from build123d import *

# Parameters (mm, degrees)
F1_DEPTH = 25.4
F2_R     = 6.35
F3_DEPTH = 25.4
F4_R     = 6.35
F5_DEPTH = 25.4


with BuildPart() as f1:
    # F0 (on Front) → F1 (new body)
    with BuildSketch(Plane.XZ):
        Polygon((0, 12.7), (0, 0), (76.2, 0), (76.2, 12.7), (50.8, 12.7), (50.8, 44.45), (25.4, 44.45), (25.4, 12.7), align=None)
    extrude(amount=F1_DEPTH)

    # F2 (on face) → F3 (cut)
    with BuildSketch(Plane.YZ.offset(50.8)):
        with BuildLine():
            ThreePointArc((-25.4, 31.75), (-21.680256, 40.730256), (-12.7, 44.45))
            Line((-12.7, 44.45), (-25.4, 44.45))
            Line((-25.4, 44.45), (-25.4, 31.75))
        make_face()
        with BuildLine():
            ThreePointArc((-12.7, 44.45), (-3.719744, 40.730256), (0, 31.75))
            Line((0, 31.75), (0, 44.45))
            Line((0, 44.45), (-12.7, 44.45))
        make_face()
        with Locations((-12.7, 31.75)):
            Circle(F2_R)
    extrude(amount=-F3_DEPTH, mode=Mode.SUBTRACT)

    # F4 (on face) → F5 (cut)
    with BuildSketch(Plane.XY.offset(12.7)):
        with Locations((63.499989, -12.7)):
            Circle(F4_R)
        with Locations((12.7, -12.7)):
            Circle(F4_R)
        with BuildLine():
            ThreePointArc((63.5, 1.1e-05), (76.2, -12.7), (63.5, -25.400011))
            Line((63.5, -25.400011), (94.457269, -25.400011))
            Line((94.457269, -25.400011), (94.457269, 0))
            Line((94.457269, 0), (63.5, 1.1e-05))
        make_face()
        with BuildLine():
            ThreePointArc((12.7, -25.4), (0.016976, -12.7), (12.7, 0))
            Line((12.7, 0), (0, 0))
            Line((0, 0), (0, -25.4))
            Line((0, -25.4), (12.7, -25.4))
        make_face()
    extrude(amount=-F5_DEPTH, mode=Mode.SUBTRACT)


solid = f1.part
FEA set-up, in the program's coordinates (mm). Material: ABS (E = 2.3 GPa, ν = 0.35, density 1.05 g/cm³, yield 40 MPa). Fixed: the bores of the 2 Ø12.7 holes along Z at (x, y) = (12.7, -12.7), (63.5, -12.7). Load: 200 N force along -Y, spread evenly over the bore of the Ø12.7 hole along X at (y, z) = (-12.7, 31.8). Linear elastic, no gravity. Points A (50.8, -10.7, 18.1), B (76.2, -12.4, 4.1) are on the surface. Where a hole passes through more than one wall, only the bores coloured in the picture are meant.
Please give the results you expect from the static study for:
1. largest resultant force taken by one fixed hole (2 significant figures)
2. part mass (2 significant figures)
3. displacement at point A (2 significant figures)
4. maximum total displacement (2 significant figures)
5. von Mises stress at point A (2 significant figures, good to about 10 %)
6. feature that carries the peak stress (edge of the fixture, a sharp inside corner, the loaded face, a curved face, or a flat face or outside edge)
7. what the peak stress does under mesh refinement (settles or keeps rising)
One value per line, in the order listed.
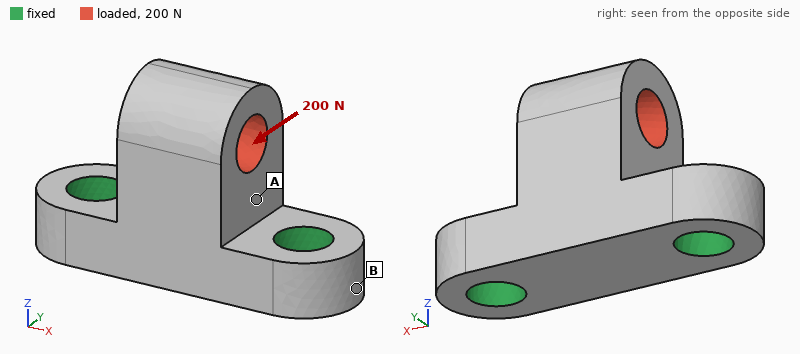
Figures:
100 N
37 g
0.038 mm
0.13 mm
1.4 MPa
edge of the fixture
keeps rising
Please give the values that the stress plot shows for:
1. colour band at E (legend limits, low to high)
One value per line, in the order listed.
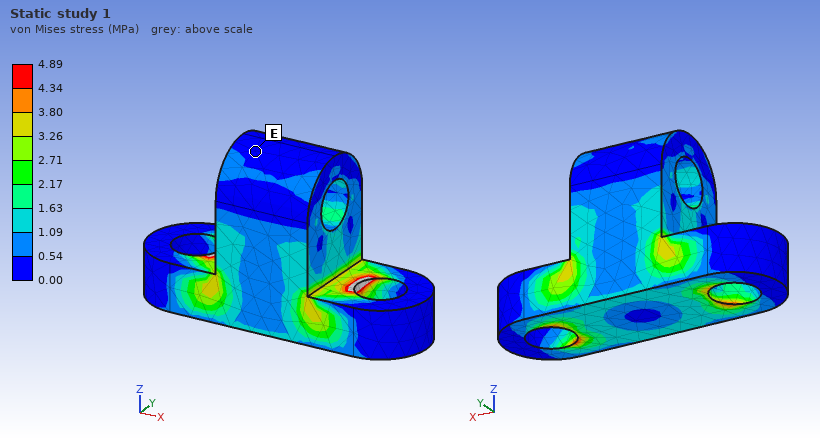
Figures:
0.00 to 0.54 MPa
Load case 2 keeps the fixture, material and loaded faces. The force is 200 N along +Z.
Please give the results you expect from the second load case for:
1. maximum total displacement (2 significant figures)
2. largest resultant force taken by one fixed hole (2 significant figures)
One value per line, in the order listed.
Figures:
14 µm
100 N
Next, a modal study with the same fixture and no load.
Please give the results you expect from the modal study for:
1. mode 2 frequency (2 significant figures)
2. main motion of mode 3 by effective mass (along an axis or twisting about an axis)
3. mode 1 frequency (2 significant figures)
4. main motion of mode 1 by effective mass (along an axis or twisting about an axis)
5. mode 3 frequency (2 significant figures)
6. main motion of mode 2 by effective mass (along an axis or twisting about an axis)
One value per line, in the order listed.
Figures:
3500 Hz
along Z
2000 Hz
along Y
5000 Hz
along X
